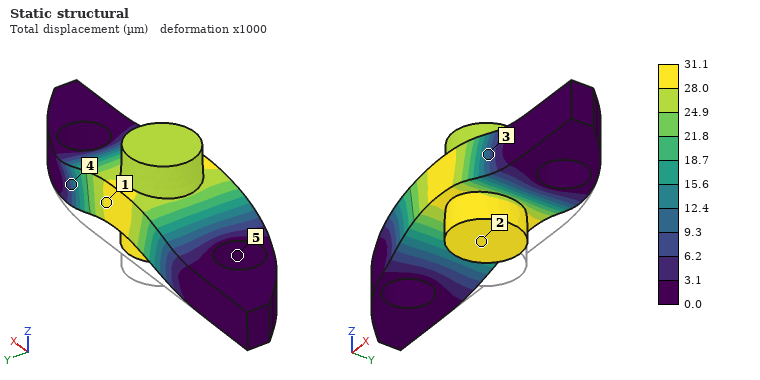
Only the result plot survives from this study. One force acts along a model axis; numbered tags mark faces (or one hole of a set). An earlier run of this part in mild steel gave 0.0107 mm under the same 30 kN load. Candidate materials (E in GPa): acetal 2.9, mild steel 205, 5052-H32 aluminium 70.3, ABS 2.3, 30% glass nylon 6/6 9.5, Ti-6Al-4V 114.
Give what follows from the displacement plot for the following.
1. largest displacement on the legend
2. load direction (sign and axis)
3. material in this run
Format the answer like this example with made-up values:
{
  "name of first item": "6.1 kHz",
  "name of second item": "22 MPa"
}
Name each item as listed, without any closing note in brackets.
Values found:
{
  "largest displacement on the legend": "31.1 µm",
  "load direction": "+Z",
  "material in this run": "5052-H32 aluminium"
}
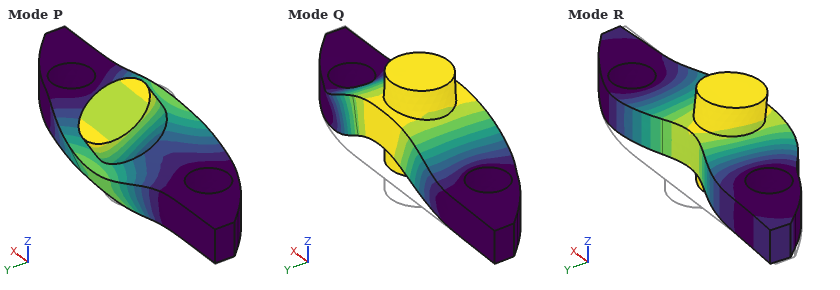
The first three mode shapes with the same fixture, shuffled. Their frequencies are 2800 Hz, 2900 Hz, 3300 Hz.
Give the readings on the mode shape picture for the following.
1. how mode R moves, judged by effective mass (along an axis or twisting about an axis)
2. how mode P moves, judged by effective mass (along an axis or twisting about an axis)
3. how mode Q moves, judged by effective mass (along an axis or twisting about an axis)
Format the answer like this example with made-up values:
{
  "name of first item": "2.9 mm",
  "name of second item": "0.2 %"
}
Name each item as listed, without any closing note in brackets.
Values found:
{
  "how mode R moves, judged by effective mass": "along Y",
  "how mode P moves, judged by effective mass": "twisting about X",
  "how mode Q moves, judged by effective mass": "along Z"
}
